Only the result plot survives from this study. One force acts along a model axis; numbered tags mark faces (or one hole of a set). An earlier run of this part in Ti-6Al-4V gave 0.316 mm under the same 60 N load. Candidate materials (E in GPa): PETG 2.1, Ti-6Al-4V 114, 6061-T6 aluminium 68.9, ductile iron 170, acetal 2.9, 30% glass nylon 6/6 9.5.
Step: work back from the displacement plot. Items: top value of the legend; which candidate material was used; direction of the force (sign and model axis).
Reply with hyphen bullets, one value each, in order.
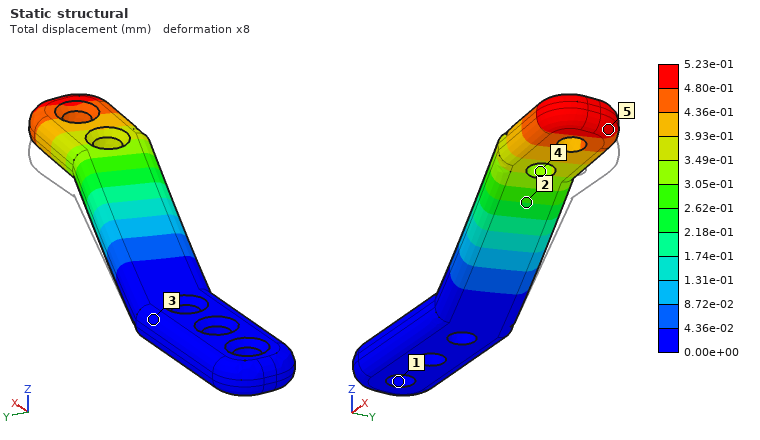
- 5.23e-01 mm
- 6061-T6 aluminium
- +Z
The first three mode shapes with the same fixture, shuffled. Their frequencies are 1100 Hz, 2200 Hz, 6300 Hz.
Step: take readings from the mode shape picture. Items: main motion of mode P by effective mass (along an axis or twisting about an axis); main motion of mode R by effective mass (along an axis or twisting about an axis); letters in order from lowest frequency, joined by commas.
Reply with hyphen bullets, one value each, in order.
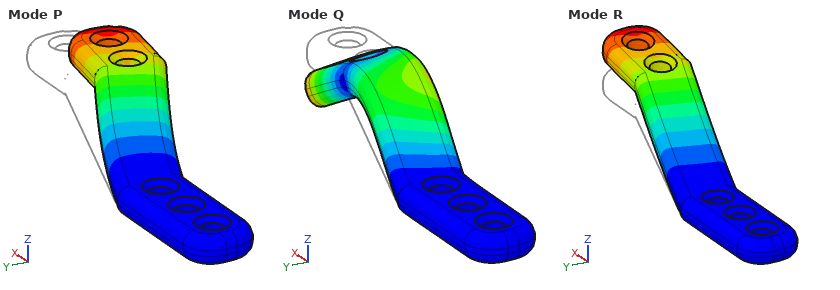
- along Y
- along Z
- R, P, Q
